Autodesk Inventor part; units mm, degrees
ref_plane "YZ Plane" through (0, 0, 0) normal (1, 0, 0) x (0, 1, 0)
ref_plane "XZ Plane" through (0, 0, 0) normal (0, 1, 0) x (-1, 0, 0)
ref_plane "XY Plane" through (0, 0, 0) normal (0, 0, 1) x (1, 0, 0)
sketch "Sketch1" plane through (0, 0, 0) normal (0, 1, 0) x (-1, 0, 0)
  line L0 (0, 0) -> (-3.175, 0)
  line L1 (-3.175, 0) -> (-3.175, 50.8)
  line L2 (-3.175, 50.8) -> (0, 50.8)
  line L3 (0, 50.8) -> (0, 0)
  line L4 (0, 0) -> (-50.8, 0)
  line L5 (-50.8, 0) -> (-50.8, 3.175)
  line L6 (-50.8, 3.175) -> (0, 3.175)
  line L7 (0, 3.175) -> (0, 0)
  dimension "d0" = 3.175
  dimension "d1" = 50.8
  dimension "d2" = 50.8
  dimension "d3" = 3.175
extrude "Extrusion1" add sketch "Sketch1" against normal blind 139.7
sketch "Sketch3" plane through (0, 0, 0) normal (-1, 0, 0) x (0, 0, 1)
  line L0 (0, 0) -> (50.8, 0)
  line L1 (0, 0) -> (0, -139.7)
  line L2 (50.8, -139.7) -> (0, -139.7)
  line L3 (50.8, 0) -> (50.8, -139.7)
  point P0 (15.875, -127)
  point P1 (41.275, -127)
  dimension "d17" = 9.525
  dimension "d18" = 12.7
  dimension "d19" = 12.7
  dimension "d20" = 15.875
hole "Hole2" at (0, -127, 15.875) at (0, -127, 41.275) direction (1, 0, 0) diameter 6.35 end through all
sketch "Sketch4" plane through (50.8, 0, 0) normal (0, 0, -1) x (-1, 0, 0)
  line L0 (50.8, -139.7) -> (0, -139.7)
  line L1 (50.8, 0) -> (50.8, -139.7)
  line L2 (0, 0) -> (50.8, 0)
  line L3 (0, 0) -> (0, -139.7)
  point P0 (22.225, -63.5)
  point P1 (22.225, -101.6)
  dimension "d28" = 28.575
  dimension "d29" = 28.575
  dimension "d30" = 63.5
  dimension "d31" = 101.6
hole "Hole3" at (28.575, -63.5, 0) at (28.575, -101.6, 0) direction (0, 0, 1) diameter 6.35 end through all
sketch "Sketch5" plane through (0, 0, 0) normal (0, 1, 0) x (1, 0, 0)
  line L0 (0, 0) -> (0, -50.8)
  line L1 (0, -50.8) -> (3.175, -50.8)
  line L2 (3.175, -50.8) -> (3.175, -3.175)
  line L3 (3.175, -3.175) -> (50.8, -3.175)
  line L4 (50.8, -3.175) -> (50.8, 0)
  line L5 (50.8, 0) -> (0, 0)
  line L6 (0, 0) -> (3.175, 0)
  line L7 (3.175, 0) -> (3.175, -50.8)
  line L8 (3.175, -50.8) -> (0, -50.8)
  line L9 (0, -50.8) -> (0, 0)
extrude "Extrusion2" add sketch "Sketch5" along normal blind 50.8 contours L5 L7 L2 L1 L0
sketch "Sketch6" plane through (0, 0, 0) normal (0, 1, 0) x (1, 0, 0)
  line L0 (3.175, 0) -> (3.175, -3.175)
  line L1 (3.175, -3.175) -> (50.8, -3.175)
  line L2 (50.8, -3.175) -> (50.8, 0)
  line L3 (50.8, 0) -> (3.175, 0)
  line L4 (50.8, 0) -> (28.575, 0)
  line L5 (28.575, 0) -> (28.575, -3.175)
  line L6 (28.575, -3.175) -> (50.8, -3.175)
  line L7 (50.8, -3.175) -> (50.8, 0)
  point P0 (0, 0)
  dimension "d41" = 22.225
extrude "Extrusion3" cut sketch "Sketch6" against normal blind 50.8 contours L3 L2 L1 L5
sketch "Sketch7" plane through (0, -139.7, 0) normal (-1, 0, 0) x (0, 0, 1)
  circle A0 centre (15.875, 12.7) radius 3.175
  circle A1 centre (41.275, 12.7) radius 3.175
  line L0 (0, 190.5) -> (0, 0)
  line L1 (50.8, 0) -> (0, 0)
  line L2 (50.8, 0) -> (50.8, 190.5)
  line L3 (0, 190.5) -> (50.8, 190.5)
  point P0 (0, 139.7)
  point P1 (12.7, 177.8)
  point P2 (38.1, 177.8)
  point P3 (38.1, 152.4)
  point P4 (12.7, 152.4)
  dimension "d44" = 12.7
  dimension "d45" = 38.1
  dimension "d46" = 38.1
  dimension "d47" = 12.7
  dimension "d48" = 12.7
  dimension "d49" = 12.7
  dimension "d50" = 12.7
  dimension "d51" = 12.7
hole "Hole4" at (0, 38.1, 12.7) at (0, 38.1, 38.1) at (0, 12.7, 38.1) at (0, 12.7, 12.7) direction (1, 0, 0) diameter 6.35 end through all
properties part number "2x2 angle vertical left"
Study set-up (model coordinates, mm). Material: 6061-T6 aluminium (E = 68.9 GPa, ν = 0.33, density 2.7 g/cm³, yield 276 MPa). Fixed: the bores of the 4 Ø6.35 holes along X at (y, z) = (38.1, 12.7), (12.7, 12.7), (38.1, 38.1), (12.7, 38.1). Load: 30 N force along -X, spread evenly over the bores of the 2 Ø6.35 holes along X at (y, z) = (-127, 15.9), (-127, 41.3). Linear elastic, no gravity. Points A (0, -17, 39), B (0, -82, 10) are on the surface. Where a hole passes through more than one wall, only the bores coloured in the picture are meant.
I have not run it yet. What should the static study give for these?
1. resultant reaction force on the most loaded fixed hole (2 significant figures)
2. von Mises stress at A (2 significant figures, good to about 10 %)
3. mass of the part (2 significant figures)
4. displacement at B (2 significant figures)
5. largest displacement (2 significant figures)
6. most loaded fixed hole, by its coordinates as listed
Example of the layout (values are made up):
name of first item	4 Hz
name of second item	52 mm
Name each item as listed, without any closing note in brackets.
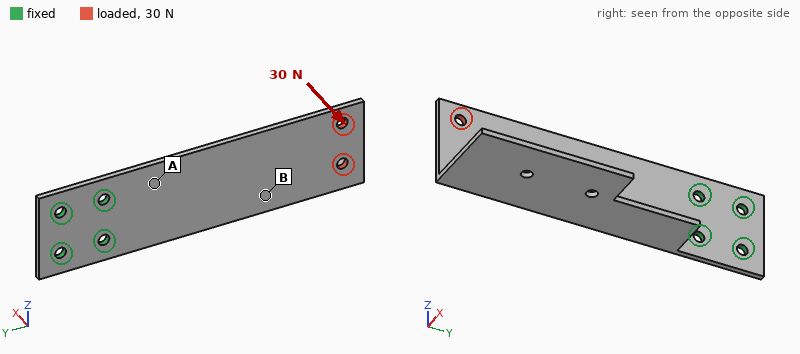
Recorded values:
resultant reaction force on the most loaded fixed hole	35 N
von Mises stress at A	18 MPa
mass of the part	130 g
displacement at B	0.78 mm
largest displacement	1.4 mm
most loaded fixed hole, by its coordinates as listed	(12.7, 12.7)
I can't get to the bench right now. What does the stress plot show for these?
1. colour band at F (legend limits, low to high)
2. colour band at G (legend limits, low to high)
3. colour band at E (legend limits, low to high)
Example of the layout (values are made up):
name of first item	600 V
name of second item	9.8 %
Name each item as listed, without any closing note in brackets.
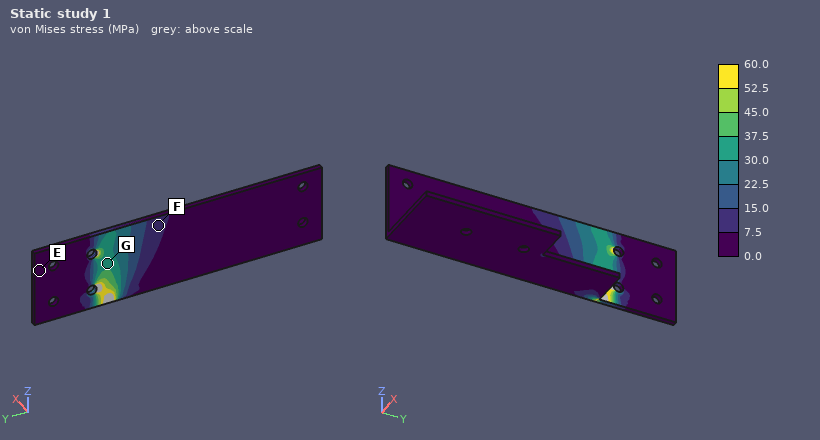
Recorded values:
colour band at F	7.5 to 15.0 MPa
colour band at G	30.0 to 37.5 MPa
colour band at E	0.0 to 7.5 MPa
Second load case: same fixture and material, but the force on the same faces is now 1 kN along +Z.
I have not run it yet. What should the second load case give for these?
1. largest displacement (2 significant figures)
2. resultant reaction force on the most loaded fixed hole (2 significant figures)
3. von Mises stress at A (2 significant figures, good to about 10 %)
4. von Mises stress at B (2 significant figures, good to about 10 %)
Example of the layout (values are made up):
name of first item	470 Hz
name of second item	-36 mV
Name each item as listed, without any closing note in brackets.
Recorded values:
largest displacement	0.54 mm
resultant reaction force on the most loaded fixed hole	3.7 kN
von Mises stress at A	40 MPa
von Mises stress at B	17 MPa
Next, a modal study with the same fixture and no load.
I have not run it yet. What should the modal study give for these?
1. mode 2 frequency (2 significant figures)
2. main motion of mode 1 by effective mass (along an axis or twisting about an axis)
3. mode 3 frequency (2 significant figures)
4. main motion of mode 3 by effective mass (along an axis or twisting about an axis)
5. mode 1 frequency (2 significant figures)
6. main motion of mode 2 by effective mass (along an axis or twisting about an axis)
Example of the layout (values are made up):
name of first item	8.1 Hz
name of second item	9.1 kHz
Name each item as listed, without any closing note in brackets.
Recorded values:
mode 2 frequency	340 Hz
main motion of mode 1 by effective mass	along X
mode 3 frequency	1100 Hz
main motion of mode 3 by effective mass	along Z
mode 1 frequency	110 Hz
main motion of mode 2 by effective mass	along Z
